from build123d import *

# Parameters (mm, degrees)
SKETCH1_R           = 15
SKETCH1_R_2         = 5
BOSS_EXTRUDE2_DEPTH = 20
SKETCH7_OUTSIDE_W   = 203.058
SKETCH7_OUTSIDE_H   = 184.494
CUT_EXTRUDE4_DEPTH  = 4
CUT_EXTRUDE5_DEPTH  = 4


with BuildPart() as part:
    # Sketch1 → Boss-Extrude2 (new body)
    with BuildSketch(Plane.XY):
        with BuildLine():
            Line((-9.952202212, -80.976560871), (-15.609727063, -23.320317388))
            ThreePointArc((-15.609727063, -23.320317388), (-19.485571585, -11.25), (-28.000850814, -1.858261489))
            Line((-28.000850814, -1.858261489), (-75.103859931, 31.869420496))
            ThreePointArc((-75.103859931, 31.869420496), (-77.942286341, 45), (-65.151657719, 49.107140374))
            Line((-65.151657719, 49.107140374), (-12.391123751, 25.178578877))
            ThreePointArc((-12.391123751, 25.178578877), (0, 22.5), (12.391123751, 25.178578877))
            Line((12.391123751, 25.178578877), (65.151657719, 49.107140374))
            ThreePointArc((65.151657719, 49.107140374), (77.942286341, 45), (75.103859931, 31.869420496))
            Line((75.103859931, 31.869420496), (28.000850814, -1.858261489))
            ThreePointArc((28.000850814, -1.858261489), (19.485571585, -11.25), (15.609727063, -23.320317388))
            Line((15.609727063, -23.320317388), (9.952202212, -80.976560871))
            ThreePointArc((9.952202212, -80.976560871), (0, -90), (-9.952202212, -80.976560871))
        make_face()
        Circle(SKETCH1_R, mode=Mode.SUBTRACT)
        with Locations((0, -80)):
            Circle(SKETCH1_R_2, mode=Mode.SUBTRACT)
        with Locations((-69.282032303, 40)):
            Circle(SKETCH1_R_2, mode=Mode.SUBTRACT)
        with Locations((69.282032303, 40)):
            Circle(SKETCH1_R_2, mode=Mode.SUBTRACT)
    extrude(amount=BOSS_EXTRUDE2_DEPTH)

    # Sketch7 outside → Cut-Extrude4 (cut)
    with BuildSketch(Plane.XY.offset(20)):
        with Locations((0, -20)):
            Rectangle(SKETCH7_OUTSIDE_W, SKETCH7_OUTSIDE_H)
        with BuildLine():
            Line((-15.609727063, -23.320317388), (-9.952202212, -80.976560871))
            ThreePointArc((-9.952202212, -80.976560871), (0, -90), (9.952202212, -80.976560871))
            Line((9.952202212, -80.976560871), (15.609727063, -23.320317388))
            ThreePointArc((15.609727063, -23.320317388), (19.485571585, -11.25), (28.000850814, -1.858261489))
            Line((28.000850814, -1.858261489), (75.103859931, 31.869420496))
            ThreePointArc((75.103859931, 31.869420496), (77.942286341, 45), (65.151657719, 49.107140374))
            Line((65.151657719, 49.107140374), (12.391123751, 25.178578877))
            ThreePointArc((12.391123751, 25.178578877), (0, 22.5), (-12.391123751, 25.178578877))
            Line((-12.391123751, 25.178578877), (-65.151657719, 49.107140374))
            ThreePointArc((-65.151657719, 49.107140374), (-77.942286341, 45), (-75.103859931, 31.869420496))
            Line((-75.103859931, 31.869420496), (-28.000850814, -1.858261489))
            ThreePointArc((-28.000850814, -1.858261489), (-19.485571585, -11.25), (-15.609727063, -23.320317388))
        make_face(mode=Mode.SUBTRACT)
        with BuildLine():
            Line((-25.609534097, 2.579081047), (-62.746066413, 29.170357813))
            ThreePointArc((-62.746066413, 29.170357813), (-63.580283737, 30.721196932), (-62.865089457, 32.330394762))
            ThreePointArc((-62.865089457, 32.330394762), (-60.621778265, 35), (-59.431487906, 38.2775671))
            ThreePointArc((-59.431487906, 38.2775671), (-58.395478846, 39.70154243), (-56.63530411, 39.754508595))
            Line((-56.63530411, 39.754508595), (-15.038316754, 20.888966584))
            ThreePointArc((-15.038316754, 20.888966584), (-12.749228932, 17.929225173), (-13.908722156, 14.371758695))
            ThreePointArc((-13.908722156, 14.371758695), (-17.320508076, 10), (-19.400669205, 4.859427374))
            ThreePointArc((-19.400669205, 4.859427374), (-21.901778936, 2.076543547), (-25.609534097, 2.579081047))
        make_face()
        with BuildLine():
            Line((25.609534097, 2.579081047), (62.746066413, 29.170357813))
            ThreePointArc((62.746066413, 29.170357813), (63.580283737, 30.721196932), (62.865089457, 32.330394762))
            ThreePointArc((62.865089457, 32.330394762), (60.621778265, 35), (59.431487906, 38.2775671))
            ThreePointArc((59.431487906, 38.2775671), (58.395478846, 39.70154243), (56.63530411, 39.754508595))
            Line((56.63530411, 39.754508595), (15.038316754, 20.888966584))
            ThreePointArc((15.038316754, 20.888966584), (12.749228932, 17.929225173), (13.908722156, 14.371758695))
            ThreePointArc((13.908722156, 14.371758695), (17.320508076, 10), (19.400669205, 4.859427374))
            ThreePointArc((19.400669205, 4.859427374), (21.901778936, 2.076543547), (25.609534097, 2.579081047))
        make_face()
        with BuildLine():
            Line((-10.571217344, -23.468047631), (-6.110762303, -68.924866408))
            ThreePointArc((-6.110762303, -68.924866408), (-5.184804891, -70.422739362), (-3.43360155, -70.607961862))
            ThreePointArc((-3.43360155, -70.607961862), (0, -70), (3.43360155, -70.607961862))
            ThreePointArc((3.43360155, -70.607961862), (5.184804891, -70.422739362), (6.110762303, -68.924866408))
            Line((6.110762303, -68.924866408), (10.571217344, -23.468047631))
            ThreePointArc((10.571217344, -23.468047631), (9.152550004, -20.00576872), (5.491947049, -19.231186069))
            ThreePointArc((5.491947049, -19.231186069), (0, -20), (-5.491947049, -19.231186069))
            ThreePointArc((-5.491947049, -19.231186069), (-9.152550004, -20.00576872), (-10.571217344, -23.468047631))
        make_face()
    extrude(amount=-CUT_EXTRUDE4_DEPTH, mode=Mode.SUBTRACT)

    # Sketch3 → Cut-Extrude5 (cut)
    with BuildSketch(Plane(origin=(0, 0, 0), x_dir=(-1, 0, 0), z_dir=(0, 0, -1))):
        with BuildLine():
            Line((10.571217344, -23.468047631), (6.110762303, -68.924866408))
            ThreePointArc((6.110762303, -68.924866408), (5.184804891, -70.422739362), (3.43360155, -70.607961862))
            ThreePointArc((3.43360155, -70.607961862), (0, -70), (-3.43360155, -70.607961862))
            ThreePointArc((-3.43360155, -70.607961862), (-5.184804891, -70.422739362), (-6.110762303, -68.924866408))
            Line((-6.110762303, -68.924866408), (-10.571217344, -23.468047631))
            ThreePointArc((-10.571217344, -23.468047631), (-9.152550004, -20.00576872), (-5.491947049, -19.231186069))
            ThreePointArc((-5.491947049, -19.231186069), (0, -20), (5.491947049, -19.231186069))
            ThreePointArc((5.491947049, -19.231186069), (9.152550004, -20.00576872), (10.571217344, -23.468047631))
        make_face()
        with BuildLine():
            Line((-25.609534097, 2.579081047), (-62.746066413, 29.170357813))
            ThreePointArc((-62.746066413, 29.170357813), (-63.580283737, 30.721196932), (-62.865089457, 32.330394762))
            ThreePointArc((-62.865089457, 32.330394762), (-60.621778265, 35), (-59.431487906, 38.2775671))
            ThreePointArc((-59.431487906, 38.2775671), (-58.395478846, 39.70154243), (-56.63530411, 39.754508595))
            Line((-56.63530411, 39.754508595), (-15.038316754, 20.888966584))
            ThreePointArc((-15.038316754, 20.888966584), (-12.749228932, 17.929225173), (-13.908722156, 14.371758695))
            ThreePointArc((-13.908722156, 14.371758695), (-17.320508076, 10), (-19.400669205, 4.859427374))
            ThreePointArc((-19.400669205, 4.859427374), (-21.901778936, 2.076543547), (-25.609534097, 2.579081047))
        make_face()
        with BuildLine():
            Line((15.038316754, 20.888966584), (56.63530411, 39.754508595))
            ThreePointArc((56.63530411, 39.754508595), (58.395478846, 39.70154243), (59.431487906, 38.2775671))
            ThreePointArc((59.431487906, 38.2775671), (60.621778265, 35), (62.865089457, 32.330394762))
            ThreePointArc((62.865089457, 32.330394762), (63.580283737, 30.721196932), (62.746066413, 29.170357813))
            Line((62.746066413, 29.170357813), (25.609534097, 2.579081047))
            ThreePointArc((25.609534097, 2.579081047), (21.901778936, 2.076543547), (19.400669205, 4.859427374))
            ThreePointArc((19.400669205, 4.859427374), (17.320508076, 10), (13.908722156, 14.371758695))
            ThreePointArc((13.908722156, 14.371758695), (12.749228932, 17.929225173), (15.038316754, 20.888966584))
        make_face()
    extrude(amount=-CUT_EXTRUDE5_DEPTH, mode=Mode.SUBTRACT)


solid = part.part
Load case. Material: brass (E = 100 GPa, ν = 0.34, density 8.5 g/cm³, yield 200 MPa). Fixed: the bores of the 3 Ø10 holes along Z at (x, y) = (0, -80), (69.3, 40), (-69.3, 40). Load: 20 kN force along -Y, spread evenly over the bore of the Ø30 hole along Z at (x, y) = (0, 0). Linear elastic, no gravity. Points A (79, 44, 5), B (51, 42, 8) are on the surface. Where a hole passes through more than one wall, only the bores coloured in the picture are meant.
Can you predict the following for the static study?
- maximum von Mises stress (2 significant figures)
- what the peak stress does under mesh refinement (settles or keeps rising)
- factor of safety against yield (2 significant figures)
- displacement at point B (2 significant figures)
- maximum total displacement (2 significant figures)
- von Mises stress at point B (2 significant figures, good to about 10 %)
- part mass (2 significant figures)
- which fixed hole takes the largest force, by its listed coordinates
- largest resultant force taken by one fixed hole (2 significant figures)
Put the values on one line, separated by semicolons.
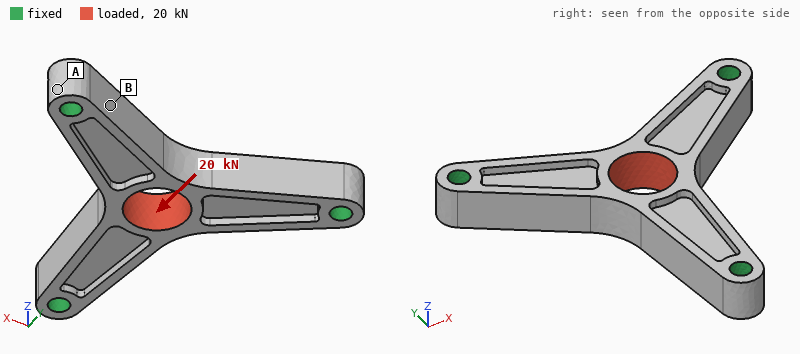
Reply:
84 MPa; settles; 2.4; 9.2 µm; 52 µm; 36 MPa; 810 g; (0, -80); 13 kN
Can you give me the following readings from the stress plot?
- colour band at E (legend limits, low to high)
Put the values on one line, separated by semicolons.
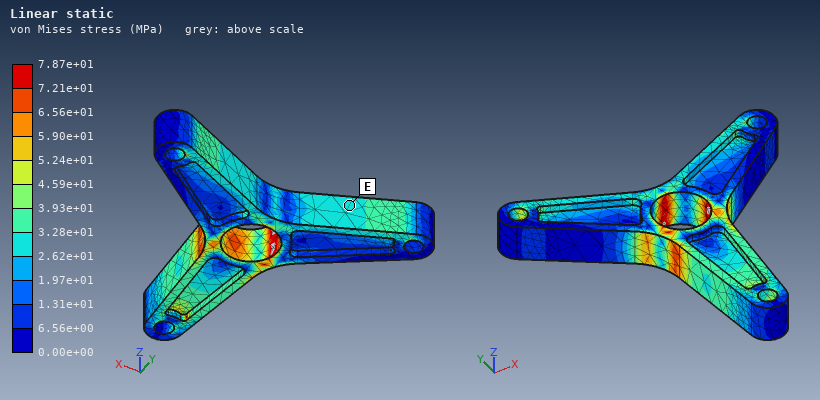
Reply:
2.62e+01 to 3.28e+01 MPa
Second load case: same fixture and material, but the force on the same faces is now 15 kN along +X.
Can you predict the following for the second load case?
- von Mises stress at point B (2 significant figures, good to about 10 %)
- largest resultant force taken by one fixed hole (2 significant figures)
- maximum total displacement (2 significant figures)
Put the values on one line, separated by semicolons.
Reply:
12 MPa; 8.4 kN; 36 µm
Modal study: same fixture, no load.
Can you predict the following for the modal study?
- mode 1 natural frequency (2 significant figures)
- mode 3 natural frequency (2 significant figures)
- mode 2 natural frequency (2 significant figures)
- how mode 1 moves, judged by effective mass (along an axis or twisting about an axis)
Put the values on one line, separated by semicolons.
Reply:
2600 Hz; 5100 Hz; 5100 Hz; along Z
